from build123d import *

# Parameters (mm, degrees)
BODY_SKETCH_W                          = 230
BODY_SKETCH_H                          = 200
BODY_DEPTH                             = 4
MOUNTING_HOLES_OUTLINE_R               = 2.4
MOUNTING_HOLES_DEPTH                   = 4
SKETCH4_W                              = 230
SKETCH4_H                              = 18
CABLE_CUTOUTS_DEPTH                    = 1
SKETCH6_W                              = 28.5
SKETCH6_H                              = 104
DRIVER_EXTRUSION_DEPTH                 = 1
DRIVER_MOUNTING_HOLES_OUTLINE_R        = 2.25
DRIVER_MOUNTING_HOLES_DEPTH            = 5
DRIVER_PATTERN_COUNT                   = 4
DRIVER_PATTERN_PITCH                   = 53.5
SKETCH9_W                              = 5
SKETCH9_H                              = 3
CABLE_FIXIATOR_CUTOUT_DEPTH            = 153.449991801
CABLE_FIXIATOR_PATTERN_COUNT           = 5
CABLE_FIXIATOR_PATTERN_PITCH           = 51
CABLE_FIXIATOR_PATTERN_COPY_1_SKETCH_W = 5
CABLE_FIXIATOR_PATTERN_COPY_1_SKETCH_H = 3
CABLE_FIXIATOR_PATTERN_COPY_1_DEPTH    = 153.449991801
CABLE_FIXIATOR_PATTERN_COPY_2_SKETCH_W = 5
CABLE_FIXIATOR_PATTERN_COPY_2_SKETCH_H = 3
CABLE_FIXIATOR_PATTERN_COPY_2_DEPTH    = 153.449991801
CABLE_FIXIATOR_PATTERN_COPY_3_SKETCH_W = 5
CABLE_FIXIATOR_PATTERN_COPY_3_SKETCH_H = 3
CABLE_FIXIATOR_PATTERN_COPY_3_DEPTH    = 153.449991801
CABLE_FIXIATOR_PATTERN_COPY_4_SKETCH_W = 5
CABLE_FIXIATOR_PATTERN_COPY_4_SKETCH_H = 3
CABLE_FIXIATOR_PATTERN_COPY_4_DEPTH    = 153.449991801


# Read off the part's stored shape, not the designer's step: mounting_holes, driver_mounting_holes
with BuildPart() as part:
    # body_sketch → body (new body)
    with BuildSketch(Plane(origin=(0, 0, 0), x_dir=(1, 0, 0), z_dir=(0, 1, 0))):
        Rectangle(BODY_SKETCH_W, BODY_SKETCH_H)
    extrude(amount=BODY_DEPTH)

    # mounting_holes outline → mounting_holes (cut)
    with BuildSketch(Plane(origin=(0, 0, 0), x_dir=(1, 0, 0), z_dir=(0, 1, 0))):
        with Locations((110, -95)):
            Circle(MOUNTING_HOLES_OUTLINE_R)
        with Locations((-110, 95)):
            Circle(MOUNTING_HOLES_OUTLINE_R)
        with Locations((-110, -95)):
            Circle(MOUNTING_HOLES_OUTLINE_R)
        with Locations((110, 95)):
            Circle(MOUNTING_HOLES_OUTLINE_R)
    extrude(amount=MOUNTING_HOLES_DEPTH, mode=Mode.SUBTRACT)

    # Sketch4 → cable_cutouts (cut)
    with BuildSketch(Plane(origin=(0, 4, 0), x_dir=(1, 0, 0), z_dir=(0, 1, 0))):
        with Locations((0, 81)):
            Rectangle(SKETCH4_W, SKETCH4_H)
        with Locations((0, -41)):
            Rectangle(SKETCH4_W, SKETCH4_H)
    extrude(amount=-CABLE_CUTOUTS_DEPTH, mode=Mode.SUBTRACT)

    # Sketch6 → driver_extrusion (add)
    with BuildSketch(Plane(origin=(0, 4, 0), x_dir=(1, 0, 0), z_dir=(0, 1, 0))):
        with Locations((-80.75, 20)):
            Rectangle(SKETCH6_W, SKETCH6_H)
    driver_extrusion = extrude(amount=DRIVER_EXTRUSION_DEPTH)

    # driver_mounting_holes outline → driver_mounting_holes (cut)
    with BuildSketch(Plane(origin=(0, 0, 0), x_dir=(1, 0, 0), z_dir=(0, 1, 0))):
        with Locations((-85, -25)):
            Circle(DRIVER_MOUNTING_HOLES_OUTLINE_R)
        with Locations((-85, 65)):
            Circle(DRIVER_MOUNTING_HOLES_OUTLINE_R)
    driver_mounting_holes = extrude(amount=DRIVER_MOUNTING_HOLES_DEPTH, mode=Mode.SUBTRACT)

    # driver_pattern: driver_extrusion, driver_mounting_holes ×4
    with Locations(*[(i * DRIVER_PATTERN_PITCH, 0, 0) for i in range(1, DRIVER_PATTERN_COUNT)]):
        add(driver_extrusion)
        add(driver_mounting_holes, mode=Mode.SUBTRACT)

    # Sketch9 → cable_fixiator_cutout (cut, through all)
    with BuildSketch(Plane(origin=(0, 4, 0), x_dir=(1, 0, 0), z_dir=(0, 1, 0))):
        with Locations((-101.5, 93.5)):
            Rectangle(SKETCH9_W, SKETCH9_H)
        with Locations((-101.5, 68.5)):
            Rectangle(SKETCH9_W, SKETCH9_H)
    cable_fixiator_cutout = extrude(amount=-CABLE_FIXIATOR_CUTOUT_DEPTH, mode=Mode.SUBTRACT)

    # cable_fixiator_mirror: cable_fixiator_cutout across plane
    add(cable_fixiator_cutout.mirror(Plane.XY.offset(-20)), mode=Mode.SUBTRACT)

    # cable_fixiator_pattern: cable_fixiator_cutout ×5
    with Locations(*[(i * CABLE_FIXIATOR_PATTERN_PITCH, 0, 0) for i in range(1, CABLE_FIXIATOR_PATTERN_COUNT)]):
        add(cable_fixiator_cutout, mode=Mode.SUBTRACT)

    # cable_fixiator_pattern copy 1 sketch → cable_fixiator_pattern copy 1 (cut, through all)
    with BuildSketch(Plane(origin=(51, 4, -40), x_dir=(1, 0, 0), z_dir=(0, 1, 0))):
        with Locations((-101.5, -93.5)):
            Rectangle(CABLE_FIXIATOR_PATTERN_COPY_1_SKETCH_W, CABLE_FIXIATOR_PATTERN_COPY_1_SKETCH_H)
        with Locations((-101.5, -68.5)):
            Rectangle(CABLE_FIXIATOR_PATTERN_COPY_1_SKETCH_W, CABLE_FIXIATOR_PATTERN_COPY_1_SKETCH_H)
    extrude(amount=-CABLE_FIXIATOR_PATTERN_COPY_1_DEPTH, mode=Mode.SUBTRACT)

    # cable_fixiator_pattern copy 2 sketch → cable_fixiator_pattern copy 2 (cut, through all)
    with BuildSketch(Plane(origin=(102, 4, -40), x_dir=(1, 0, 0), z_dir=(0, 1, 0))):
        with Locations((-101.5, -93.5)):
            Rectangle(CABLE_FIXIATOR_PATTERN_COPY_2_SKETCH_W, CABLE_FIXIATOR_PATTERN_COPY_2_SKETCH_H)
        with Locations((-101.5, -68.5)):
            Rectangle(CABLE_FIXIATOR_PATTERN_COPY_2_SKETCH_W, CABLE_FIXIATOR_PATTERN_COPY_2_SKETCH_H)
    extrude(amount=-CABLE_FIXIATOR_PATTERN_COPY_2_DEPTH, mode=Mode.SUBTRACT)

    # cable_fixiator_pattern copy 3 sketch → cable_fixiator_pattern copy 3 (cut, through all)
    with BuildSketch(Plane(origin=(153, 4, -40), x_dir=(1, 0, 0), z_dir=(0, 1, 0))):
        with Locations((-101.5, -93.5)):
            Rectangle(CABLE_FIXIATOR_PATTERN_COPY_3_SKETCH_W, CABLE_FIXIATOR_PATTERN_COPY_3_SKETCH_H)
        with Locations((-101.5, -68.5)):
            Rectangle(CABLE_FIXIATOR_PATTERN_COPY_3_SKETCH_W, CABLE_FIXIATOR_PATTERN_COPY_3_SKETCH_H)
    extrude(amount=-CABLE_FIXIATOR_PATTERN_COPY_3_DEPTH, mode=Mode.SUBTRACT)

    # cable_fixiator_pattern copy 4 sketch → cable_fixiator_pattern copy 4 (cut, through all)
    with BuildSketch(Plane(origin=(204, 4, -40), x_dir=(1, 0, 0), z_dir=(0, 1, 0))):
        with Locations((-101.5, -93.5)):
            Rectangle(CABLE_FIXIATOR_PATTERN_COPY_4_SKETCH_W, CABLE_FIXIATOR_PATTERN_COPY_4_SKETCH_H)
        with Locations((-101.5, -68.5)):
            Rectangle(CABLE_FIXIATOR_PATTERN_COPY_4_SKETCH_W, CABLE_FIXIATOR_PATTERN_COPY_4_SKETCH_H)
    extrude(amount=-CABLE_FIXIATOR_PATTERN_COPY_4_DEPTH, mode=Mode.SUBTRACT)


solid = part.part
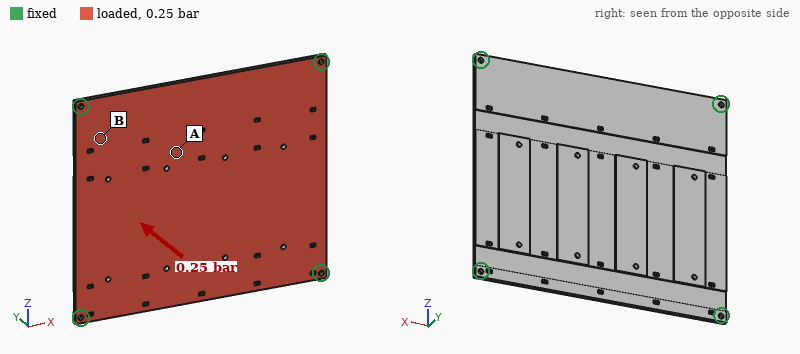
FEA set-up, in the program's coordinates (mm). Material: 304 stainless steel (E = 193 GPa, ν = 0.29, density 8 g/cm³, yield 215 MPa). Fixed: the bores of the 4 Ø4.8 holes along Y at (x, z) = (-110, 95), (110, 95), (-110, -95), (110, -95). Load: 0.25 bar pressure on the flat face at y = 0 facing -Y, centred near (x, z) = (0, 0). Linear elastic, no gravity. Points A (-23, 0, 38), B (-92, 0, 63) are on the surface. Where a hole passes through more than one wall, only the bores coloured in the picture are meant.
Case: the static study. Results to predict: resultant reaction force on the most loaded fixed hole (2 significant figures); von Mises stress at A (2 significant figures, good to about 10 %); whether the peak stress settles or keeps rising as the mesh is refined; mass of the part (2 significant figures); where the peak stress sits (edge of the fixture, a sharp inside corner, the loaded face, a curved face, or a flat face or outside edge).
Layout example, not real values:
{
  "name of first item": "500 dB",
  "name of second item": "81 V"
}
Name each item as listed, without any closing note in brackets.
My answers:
{
  "resultant reaction force on the most loaded fixed hole": "340 N",
  "von Mises stress at A": "30 MPa",
  "whether the peak stress settles or keeps rising as the mesh is refined": "keeps rising",
  "mass of the part": "1.5 kg",
  "where the peak stress sits": "edge of the fixture"
}
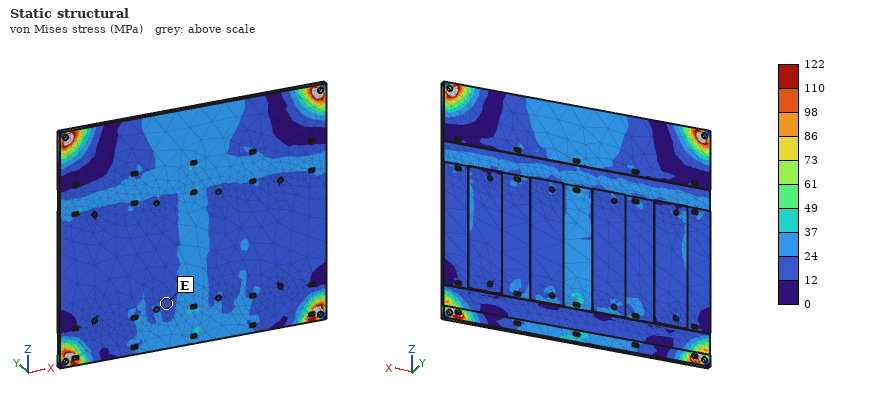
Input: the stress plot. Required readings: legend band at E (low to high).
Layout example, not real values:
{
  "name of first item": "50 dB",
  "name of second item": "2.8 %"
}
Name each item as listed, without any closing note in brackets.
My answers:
{
  "legend band at E": "12 to 24 MPa"
}
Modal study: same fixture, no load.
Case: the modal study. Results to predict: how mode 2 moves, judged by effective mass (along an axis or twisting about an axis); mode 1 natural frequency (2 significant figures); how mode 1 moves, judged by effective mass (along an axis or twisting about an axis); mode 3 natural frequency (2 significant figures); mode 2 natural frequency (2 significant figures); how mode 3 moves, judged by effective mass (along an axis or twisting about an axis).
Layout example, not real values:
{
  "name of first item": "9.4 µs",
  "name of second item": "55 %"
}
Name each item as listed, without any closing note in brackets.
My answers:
{
  "how mode 2 moves, judged by effective mass": "twisting about X",
  "mode 1 natural frequency": "250 Hz",
  "how mode 1 moves, judged by effective mass": "along Y",
  "mode 3 natural frequency": "510 Hz",
  "mode 2 natural frequency": "470 Hz",
  "how mode 3 moves, judged by effective mass": "twisting about Z"
}
